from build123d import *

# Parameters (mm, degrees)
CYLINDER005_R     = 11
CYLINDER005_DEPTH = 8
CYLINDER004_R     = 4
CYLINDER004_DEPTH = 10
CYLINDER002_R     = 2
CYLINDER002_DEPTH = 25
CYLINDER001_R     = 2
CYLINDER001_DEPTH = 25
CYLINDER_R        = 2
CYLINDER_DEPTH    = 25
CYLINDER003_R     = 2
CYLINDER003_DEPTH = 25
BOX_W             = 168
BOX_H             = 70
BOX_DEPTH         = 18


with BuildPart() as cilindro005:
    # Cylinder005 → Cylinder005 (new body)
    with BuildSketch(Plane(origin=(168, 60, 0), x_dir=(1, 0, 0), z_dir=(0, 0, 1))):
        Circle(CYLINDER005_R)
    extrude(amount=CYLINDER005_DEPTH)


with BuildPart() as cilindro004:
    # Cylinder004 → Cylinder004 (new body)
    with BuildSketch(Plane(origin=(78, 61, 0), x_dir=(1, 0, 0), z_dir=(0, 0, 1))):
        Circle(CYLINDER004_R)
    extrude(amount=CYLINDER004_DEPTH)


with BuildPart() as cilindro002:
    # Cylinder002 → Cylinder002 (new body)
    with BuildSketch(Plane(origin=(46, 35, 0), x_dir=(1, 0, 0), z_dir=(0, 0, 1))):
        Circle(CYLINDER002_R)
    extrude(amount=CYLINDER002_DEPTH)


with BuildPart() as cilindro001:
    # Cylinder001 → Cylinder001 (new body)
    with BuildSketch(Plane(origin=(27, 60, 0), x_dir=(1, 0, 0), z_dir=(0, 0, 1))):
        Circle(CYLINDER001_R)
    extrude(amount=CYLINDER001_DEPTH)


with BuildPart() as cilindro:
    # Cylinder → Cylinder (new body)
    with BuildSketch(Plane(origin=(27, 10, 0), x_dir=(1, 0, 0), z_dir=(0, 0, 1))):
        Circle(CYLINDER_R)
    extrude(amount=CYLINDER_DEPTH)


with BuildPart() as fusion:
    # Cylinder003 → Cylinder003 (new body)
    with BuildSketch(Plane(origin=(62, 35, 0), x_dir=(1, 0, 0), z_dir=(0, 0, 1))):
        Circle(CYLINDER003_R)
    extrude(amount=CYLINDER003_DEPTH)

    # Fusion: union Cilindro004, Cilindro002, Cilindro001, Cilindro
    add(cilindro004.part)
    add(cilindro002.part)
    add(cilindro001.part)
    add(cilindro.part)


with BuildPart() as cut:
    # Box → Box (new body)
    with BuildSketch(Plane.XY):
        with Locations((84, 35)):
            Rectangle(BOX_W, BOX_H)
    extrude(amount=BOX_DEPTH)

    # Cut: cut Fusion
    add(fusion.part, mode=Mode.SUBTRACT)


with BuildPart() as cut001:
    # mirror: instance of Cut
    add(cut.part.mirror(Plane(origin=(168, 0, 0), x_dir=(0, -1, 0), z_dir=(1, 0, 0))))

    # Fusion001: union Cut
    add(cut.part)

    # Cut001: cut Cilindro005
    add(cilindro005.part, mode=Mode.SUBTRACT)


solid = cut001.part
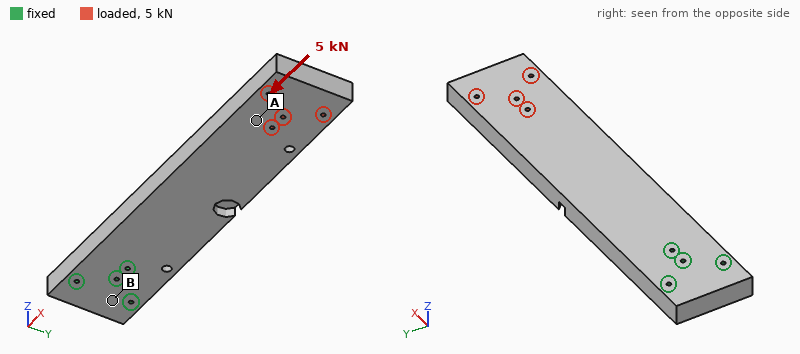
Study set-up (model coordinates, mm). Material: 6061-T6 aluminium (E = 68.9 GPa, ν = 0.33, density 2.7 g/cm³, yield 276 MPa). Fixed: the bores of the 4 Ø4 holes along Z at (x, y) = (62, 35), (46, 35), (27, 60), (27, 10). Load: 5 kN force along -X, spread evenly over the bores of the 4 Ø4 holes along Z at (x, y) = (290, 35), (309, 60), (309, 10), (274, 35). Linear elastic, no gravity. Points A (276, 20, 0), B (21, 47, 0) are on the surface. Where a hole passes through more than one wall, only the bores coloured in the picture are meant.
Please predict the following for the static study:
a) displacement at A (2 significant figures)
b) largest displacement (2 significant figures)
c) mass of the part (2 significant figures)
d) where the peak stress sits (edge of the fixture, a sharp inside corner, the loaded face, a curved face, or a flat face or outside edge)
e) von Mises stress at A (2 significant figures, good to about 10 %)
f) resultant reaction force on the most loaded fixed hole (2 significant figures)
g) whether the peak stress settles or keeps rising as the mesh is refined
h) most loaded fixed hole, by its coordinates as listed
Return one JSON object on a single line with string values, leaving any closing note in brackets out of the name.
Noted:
{"displacement at A": "19 µm", "largest displacement": "26 µm", "mass of the part": "1.1 kg", "where the peak stress sits": "edge of the fixture", "von Mises stress at A": "3.4 MPa", "resultant reaction force on the most loaded fixed hole": "2.3 kN", "whether the peak stress settles or keeps rising as the mesh is refined": "keeps rising", "most loaded fixed hole, by its coordinates as listed": "(62, 35)"}
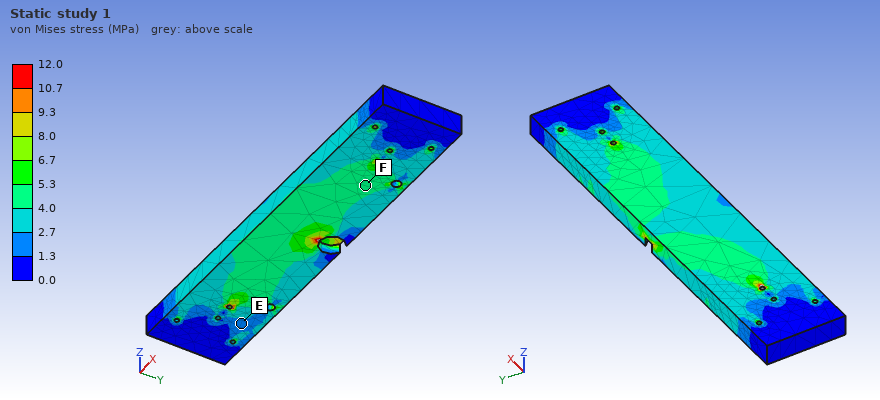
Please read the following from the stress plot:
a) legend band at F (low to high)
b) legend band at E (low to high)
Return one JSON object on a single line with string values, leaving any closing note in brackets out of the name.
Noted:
{"legend band at F": "4.0 to 5.3 MPa", "legend band at E": "1.3 to 2.7 MPa"}
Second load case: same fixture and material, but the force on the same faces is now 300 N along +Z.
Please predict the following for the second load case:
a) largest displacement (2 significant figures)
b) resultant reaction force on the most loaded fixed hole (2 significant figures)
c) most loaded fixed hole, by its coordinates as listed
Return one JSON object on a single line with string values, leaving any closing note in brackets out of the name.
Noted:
{"largest displacement": "0.78 mm", "resultant reaction force on the most loaded fixed hole": "1.8 kN", "most loaded fixed hole, by its coordinates as listed": "(62, 35)"}
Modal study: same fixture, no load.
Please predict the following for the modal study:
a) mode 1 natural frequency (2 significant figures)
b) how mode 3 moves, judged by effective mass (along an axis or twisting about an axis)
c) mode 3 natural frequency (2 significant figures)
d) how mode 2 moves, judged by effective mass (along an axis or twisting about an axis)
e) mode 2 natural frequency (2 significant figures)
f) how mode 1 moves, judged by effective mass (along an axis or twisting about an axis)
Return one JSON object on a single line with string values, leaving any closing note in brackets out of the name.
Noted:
{"mode 1 natural frequency": "180 Hz", "how mode 3 moves, judged by effective mass": "along Z", "mode 3 natural frequency": "1100 Hz", "how mode 2 moves, judged by effective mass": "along Y", "mode 2 natural frequency": "590 Hz", "how mode 1 moves, judged by effective mass": "along Z"}
